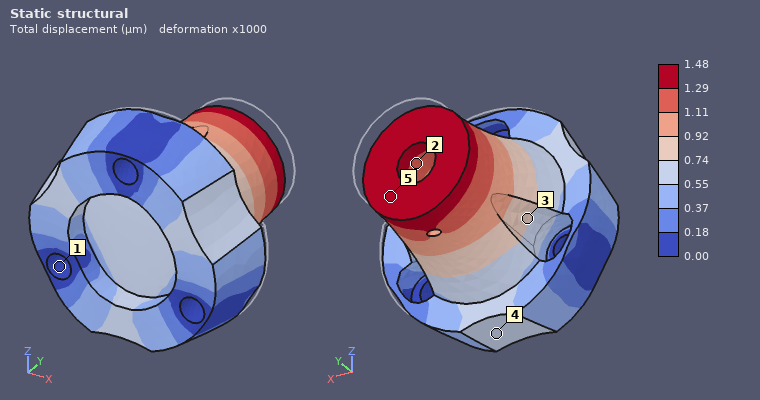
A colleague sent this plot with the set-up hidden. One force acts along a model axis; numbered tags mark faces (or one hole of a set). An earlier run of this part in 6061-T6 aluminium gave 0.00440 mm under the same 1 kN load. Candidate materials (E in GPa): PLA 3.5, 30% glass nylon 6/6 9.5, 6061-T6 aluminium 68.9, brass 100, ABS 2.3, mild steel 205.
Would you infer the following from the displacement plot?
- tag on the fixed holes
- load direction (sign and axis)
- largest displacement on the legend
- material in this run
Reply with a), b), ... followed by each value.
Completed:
a) 1
b) -Y
c) 1.48 µm
d) mild steel
